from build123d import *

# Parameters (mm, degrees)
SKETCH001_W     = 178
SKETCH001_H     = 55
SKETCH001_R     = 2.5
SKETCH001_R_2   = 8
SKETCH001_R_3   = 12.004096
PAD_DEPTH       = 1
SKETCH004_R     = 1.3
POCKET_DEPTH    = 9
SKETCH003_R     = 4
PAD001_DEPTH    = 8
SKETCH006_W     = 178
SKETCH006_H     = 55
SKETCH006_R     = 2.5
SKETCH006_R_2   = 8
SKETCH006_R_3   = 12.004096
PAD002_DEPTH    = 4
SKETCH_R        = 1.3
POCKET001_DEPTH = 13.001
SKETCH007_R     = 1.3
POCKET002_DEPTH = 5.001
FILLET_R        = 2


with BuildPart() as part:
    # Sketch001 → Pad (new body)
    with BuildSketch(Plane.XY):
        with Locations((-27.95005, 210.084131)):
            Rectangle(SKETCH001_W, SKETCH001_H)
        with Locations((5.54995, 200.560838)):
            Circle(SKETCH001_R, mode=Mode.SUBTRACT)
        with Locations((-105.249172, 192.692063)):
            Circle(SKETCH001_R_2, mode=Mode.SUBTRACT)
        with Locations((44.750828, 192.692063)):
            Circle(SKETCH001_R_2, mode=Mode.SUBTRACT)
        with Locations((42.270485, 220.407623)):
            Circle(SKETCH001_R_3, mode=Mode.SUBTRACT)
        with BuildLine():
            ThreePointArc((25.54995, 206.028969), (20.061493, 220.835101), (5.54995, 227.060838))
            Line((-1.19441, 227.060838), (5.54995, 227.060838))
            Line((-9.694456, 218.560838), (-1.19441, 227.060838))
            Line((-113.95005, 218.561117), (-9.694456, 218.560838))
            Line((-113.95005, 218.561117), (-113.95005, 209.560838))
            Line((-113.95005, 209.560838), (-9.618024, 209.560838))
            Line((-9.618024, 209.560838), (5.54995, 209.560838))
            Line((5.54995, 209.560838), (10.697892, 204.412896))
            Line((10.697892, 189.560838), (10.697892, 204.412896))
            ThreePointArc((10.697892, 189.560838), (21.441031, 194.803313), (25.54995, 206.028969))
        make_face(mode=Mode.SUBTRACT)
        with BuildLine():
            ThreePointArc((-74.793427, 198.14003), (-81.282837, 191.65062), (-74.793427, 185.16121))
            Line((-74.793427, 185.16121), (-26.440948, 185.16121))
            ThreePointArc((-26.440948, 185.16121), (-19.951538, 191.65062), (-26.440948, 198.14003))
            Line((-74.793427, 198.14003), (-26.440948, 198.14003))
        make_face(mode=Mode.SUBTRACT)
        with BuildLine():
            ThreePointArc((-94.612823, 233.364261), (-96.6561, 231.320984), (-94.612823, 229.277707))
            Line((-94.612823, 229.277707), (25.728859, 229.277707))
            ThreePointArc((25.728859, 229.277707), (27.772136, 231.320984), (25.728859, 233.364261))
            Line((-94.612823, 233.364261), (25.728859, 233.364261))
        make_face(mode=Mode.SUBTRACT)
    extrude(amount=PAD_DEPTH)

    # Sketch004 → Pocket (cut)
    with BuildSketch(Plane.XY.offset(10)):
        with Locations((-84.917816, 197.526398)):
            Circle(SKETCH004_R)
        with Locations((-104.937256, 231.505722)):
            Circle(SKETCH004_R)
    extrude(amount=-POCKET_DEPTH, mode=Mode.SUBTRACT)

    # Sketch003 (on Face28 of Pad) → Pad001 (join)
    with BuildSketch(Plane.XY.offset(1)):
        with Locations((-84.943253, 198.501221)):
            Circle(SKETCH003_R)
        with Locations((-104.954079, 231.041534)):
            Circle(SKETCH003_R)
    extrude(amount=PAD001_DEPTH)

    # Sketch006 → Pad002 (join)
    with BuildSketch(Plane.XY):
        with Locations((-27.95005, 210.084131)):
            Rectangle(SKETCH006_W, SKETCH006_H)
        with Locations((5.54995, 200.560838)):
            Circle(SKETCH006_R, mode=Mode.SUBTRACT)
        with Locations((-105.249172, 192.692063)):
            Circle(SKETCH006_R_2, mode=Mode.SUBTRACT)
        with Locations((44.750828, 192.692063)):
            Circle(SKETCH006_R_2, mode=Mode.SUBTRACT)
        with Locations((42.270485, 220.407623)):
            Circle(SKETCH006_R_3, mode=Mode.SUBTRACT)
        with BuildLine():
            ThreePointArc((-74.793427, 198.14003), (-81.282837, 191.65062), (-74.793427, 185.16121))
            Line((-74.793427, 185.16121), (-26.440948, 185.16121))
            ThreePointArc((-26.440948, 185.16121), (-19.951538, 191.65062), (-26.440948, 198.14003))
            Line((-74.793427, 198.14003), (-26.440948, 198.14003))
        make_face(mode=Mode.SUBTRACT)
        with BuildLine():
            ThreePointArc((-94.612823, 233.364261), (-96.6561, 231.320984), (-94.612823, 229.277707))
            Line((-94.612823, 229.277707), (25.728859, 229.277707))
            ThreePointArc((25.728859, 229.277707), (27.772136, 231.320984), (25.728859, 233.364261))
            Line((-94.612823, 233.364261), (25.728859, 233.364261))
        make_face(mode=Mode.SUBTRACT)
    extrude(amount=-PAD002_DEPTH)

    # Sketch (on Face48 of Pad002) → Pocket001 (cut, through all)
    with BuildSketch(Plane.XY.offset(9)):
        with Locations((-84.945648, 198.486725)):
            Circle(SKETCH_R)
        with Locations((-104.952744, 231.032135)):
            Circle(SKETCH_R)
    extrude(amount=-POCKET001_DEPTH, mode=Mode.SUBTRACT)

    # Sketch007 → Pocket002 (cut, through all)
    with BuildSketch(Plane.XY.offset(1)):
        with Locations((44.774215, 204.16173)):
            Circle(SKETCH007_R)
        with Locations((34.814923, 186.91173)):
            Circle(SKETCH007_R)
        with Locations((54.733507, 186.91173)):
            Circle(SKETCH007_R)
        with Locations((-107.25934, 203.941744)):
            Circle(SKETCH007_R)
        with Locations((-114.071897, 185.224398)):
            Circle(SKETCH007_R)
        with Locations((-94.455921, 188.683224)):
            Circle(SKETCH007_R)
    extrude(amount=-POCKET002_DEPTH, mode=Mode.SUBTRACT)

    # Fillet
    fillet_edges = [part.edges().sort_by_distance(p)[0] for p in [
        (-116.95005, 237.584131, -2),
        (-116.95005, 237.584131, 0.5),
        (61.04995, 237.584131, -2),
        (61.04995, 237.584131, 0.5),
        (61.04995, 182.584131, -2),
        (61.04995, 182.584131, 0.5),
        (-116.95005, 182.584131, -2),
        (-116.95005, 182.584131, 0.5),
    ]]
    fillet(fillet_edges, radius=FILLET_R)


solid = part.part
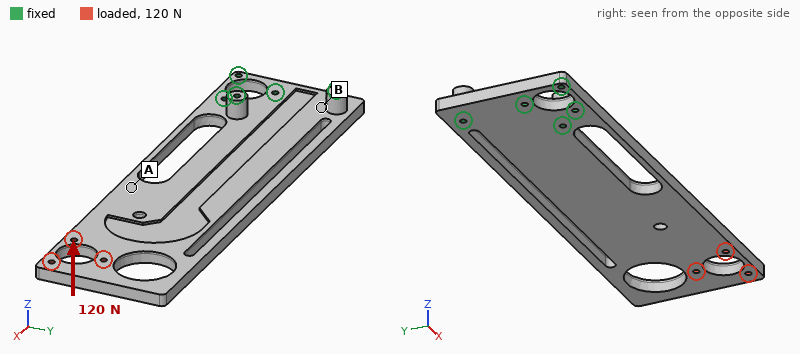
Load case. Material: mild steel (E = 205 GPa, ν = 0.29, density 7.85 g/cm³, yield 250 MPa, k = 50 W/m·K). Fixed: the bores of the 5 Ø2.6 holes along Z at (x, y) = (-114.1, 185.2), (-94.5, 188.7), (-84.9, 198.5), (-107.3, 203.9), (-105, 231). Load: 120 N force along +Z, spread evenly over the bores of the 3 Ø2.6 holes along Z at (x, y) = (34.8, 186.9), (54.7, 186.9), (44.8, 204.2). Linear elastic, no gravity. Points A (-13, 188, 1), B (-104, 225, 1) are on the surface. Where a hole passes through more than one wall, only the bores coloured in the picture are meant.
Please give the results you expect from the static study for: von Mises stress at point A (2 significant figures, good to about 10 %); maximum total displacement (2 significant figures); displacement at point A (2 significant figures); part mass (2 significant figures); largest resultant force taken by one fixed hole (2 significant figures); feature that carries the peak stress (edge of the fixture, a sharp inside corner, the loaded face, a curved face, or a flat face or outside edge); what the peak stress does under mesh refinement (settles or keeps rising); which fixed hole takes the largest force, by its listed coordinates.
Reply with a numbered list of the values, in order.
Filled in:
1. 25 MPa
2. 1.5 mm
3. 0.52 mm
4. 290 g
5. 600 N
6. edge of the fixture
7. keeps rising
8. (-84.9, 198.5)
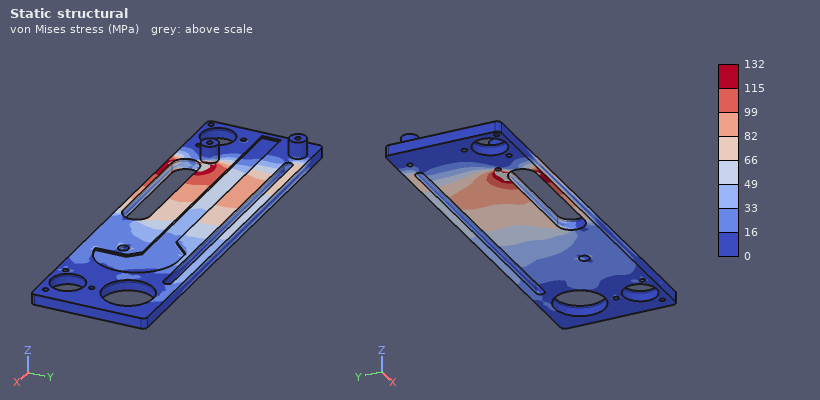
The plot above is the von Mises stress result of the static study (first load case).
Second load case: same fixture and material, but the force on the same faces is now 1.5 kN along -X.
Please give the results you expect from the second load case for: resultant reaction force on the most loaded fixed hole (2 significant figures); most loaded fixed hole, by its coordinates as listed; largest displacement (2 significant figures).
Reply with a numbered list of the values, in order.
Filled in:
1. 850 N
2. (-84.9, 198.5)
3. 52 µm
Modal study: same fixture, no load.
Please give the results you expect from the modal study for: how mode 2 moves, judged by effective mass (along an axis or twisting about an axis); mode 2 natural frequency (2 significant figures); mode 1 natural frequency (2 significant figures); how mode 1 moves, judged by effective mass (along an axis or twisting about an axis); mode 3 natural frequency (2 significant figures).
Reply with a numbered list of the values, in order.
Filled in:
1. twisting about X
2. 810 Hz
3. 170 Hz
4. along Z
5. 1100 Hz
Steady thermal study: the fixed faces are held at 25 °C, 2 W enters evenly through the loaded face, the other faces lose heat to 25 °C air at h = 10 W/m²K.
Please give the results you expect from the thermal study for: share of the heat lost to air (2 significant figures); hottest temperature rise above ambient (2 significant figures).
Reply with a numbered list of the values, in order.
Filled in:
1. 64 %
2. 20 K
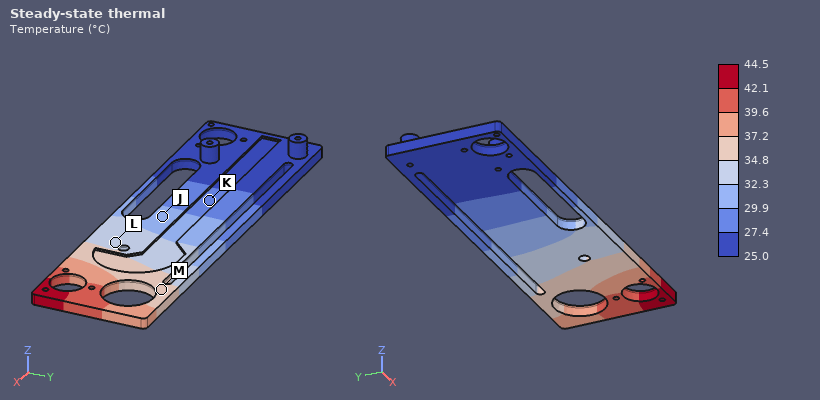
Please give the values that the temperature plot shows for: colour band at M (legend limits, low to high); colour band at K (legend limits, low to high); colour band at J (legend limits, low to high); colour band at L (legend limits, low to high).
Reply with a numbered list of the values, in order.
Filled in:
1. 34.8 to 37.2 °C
2. 27.4 to 29.9 °C
3. 29.9 to 32.3 °C
4. 32.3 to 34.8 °C
